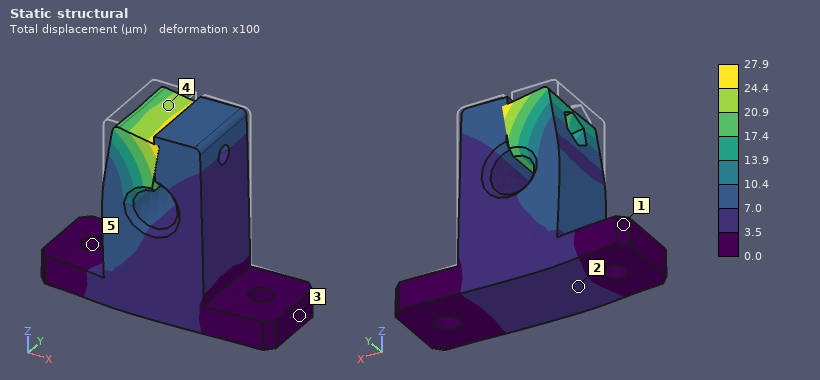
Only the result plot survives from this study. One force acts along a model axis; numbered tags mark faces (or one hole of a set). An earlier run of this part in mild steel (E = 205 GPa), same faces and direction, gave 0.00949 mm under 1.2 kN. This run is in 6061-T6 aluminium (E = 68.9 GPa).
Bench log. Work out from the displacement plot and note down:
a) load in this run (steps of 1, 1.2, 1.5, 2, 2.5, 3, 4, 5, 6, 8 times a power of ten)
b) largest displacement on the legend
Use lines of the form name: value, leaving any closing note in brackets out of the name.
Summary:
load in this run: 1.2 kN
largest displacement on the legend: 27.9 µm
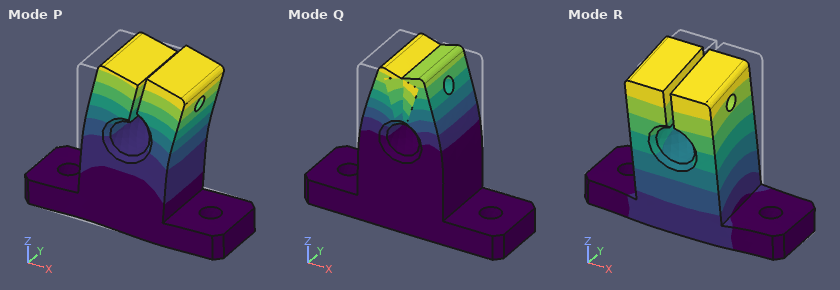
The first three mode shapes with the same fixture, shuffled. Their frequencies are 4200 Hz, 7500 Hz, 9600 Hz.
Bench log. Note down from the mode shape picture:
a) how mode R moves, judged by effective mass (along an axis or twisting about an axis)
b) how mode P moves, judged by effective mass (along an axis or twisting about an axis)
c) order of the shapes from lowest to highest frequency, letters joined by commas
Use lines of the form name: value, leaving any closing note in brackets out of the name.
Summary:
how mode R moves, judged by effective mass: along Y
how mode P moves, judged by effective mass: along X
order of the shapes from lowest to highest frequency, letters joined by commas: R, P, Q
